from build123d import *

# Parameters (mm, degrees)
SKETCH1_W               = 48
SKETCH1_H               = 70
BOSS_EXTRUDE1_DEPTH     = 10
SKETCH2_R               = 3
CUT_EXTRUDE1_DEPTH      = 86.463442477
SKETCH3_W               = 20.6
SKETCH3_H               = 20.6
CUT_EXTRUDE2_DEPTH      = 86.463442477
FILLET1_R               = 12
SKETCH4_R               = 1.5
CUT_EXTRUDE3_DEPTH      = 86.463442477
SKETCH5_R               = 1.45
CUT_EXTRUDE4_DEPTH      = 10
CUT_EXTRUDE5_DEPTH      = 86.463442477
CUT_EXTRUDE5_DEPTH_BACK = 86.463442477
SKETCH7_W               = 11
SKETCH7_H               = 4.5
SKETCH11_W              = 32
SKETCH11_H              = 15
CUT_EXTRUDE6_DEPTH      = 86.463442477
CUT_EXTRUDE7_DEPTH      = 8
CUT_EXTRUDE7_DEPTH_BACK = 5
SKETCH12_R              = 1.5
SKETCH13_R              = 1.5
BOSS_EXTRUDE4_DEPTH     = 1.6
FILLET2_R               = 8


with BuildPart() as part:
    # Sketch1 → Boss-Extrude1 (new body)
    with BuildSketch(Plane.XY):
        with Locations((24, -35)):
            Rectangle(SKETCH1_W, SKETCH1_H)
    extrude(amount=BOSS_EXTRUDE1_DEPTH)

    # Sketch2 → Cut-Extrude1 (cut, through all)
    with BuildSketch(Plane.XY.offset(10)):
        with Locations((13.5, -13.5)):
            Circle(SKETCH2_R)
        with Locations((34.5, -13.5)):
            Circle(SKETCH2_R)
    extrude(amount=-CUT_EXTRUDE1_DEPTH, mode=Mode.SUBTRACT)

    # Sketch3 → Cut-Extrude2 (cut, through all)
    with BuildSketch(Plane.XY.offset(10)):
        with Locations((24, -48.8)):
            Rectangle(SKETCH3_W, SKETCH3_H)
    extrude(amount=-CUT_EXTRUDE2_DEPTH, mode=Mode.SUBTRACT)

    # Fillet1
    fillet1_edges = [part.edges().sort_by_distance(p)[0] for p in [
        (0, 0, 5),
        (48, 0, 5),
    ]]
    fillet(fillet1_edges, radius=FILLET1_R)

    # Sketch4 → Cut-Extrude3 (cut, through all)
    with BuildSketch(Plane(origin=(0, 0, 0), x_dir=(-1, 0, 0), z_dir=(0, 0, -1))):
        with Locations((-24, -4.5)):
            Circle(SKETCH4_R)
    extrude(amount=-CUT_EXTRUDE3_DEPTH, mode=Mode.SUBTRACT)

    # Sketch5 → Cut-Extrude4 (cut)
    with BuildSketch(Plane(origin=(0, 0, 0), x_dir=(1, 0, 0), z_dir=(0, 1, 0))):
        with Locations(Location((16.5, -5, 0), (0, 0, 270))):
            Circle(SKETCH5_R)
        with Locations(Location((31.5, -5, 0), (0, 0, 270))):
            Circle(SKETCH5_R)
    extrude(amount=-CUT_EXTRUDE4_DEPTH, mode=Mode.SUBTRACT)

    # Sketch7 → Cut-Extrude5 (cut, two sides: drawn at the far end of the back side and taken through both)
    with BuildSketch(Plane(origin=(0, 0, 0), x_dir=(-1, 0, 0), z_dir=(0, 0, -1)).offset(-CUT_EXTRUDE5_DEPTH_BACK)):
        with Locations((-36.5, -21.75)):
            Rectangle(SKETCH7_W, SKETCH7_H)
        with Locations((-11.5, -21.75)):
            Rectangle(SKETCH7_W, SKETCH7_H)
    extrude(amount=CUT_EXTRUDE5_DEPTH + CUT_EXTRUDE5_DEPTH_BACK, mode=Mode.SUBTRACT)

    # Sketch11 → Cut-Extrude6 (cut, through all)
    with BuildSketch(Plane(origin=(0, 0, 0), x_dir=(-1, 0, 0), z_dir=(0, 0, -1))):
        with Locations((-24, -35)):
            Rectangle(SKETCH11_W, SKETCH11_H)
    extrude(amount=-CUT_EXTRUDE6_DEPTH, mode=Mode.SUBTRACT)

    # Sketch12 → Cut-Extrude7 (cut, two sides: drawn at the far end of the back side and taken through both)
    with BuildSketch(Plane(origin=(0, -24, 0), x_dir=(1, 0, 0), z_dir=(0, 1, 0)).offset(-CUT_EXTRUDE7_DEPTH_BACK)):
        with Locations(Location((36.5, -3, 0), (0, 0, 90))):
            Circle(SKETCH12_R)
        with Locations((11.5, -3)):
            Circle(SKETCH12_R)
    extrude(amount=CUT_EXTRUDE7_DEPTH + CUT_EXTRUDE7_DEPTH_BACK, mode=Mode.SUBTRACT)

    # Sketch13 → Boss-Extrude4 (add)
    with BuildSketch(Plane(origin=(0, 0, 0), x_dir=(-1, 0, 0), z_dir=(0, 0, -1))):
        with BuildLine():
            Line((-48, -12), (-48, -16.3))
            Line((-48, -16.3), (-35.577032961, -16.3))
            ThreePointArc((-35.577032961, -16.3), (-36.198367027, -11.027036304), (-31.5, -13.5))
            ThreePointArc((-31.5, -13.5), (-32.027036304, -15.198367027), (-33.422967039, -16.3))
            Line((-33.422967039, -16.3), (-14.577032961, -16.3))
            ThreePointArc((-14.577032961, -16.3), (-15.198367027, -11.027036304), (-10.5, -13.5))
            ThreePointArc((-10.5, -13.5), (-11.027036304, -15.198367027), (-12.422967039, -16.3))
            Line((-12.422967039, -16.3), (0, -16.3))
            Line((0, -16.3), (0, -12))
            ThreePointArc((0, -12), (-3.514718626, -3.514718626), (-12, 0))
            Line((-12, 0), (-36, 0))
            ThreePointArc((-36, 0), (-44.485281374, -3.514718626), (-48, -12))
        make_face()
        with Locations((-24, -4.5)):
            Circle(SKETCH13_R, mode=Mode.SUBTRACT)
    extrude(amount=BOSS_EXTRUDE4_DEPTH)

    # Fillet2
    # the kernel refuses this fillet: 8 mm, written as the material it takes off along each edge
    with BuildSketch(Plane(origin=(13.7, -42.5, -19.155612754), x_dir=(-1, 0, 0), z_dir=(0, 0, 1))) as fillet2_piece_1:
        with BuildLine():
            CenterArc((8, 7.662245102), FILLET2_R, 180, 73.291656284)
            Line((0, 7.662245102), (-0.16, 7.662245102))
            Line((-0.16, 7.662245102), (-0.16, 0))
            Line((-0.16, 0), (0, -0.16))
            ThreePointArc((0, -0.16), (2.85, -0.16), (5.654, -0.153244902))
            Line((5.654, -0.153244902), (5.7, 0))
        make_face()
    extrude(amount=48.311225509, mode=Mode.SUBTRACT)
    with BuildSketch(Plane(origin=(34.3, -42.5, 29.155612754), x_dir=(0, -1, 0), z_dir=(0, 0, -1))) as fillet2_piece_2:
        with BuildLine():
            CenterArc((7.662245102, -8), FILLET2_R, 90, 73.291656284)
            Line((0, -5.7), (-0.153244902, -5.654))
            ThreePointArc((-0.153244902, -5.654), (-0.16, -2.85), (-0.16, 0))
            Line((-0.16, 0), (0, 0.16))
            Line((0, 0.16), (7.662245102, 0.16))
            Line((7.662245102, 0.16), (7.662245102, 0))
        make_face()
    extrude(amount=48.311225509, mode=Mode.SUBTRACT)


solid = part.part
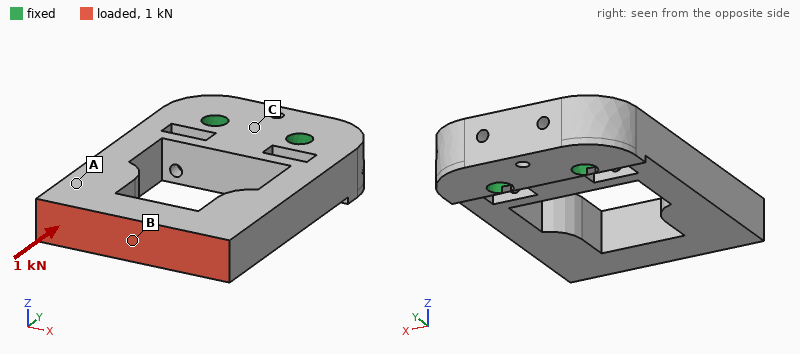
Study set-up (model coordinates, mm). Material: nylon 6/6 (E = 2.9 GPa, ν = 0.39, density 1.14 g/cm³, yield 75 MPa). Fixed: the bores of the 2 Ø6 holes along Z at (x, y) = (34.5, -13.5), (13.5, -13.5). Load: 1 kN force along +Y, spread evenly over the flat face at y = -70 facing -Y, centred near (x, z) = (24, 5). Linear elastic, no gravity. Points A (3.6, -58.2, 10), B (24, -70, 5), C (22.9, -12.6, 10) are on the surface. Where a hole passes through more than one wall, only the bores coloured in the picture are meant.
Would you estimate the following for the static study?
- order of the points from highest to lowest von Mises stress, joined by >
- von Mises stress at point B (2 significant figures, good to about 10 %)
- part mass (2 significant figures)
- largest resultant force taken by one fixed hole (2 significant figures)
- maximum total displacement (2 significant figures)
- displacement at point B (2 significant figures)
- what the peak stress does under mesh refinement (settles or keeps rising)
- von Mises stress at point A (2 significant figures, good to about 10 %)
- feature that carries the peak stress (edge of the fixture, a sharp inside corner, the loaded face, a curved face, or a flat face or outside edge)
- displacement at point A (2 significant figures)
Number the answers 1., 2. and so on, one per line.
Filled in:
1. B > A > C
2. 7.0 MPa
3. 27 g
4. 510 N
5. 0.21 mm
6. 0.20 mm
7. keeps rising
8. 2.8 MPa
9. edge of the fixture
10. 0.13 mm
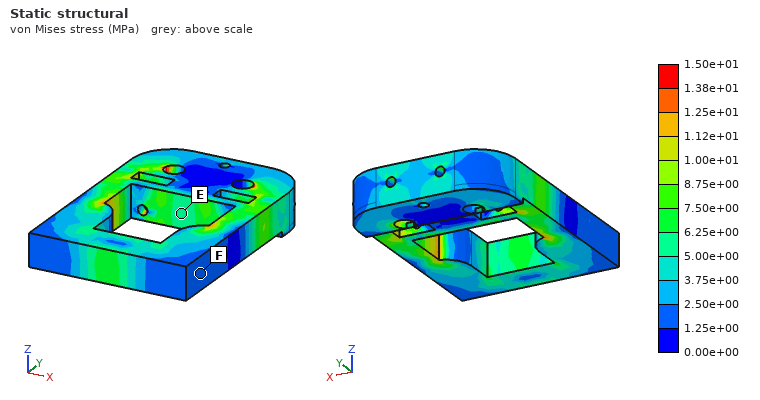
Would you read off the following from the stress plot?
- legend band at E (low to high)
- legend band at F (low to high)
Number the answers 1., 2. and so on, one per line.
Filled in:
1. 5.00e+00 to 6.25e+00 MPa
2. 1.25e+00 to 2.50e+00 MPa
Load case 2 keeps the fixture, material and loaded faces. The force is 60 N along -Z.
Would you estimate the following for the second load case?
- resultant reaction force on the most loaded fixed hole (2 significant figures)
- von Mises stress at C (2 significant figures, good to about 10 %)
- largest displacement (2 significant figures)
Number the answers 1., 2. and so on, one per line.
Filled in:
1. 31 N
2. 1.1 MPa
3. 0.99 mm
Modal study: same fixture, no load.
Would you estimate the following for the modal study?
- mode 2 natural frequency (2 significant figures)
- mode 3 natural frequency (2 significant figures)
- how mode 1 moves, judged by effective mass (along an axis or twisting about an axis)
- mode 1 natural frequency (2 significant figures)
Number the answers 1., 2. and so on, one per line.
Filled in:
1. 1200 Hz
2. 1200 Hz
3. along Z
4. 500 Hz
